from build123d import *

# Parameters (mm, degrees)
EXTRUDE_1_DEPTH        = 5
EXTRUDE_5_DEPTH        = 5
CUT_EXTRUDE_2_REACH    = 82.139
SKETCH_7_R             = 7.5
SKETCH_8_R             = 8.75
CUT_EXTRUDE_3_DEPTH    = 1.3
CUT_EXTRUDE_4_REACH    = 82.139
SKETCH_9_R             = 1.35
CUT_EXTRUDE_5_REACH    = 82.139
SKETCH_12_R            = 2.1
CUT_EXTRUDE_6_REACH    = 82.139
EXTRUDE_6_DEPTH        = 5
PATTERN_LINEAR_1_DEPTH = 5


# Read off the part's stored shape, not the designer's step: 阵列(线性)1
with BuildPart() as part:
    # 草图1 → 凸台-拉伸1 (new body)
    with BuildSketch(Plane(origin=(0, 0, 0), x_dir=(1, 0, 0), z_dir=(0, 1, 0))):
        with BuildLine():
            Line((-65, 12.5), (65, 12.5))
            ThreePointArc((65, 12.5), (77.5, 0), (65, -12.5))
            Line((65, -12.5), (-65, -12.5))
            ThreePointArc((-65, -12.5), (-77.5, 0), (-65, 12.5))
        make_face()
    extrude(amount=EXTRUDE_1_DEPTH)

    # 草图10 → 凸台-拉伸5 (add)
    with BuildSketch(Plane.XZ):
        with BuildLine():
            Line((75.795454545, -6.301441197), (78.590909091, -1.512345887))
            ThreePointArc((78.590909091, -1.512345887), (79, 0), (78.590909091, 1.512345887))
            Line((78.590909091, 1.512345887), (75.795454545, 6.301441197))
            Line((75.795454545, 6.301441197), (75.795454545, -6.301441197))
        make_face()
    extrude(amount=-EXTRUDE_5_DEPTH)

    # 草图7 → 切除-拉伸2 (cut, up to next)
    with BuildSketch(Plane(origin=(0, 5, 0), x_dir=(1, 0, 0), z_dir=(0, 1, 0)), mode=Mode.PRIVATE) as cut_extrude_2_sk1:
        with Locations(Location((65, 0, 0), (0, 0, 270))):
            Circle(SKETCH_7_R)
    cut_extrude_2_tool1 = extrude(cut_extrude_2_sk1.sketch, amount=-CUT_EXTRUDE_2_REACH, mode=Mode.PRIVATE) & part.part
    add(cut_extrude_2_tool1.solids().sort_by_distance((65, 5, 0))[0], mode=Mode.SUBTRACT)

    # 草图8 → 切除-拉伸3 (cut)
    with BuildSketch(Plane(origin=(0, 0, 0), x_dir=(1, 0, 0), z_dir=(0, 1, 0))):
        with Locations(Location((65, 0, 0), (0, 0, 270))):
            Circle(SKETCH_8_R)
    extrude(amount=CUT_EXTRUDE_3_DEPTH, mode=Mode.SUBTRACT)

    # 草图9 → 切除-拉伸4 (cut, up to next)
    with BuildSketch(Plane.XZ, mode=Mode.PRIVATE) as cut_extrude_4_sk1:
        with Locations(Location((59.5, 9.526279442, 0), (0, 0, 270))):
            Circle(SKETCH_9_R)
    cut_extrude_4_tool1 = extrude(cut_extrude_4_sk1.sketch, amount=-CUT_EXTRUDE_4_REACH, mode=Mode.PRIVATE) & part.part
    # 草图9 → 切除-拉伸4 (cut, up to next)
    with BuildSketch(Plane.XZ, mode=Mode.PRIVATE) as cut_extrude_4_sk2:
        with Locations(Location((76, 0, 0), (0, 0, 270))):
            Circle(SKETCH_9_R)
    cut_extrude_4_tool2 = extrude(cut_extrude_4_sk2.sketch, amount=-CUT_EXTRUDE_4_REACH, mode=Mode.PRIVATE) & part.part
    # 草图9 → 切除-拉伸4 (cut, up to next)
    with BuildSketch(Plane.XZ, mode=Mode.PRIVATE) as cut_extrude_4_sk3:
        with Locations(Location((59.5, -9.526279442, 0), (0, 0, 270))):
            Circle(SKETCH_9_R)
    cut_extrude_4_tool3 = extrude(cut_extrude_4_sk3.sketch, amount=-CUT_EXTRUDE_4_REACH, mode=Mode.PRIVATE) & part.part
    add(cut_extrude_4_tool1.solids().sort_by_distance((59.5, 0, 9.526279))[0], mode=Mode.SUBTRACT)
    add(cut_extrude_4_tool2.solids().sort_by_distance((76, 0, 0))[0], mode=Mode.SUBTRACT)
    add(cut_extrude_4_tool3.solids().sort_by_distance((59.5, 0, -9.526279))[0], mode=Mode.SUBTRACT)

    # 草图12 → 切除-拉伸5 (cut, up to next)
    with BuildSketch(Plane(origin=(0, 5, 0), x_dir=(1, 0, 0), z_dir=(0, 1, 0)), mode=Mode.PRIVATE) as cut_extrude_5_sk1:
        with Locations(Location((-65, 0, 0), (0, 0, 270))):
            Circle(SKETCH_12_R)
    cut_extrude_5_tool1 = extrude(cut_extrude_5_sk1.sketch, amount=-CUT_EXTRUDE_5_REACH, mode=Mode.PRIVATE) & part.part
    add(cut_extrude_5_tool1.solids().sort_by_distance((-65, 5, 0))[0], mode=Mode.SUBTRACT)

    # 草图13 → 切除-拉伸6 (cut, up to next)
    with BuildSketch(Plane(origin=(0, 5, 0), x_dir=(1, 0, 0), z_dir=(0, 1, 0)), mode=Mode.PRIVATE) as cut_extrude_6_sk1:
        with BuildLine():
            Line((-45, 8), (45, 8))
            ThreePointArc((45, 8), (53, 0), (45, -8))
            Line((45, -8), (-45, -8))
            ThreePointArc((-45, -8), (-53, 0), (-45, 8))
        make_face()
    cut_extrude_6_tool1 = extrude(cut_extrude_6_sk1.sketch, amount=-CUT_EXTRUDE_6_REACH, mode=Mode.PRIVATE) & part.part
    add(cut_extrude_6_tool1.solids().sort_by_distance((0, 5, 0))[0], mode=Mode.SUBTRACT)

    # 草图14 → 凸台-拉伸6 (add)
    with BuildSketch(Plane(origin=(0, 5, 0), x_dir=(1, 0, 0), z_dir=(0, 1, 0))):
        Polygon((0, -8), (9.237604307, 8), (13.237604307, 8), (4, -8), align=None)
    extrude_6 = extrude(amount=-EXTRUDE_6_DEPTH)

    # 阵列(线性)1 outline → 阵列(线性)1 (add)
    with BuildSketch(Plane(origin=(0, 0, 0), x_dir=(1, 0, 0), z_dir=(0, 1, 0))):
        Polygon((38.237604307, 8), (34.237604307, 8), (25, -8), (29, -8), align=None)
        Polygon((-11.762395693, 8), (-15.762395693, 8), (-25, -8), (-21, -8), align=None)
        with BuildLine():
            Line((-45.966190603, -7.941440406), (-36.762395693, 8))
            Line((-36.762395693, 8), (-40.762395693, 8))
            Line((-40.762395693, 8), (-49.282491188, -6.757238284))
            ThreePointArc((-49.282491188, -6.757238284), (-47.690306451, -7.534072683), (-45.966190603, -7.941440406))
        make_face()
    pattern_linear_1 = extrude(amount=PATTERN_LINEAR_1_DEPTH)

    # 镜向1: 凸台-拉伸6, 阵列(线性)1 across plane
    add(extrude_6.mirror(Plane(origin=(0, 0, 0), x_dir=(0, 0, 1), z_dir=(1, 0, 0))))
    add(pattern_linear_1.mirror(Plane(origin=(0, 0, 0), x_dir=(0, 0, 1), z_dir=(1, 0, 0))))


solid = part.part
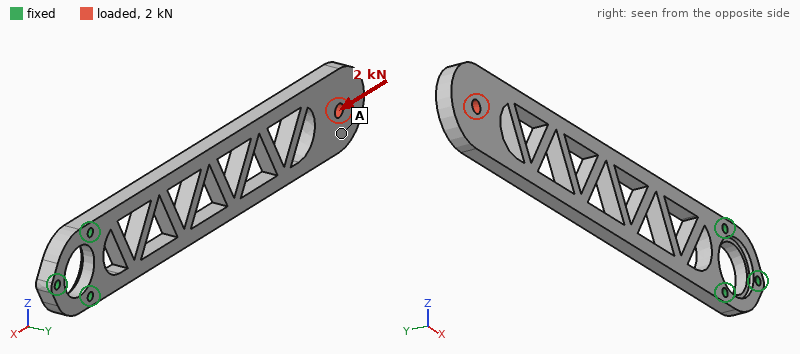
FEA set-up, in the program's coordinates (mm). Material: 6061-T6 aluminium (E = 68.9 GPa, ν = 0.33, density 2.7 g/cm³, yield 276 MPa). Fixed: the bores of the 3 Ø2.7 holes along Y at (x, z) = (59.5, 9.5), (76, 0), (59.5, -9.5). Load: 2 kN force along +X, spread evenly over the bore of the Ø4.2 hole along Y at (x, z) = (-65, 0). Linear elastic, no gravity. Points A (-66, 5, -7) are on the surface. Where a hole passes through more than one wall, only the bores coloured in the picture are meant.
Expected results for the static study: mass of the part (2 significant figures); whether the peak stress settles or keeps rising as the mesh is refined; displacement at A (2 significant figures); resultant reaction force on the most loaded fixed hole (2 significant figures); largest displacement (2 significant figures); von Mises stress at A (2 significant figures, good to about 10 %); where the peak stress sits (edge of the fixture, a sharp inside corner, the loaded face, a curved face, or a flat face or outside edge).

32 g
keeps rising
71 µm
1000 N
75 µm
13 MPa
a sharp inside corner
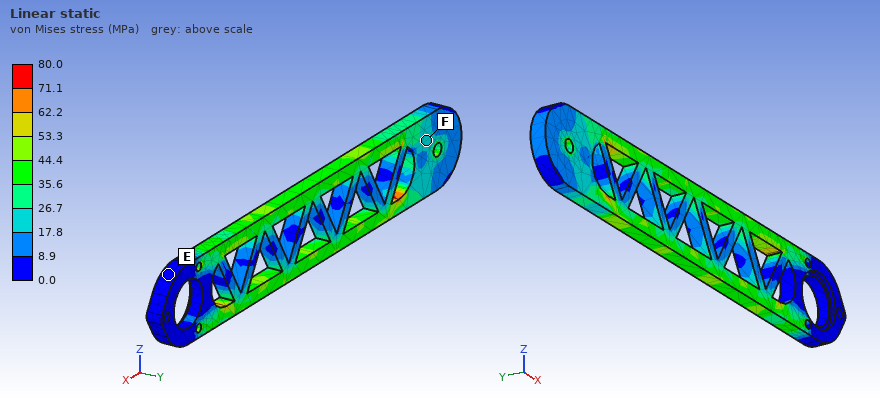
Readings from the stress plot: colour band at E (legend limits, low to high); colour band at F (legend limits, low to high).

0.0 to 8.9 MPa
17.8 to 26.7 MPa
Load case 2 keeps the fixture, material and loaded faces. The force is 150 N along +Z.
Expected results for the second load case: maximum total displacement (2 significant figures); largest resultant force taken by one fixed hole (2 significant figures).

0.35 mm
930 N
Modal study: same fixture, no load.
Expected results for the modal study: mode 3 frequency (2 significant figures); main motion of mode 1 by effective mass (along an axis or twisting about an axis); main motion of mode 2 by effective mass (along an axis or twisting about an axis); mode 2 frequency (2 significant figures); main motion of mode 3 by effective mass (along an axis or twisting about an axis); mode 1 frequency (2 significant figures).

1200 Hz
along Y
along Z
1000 Hz
along Y
170 Hz
